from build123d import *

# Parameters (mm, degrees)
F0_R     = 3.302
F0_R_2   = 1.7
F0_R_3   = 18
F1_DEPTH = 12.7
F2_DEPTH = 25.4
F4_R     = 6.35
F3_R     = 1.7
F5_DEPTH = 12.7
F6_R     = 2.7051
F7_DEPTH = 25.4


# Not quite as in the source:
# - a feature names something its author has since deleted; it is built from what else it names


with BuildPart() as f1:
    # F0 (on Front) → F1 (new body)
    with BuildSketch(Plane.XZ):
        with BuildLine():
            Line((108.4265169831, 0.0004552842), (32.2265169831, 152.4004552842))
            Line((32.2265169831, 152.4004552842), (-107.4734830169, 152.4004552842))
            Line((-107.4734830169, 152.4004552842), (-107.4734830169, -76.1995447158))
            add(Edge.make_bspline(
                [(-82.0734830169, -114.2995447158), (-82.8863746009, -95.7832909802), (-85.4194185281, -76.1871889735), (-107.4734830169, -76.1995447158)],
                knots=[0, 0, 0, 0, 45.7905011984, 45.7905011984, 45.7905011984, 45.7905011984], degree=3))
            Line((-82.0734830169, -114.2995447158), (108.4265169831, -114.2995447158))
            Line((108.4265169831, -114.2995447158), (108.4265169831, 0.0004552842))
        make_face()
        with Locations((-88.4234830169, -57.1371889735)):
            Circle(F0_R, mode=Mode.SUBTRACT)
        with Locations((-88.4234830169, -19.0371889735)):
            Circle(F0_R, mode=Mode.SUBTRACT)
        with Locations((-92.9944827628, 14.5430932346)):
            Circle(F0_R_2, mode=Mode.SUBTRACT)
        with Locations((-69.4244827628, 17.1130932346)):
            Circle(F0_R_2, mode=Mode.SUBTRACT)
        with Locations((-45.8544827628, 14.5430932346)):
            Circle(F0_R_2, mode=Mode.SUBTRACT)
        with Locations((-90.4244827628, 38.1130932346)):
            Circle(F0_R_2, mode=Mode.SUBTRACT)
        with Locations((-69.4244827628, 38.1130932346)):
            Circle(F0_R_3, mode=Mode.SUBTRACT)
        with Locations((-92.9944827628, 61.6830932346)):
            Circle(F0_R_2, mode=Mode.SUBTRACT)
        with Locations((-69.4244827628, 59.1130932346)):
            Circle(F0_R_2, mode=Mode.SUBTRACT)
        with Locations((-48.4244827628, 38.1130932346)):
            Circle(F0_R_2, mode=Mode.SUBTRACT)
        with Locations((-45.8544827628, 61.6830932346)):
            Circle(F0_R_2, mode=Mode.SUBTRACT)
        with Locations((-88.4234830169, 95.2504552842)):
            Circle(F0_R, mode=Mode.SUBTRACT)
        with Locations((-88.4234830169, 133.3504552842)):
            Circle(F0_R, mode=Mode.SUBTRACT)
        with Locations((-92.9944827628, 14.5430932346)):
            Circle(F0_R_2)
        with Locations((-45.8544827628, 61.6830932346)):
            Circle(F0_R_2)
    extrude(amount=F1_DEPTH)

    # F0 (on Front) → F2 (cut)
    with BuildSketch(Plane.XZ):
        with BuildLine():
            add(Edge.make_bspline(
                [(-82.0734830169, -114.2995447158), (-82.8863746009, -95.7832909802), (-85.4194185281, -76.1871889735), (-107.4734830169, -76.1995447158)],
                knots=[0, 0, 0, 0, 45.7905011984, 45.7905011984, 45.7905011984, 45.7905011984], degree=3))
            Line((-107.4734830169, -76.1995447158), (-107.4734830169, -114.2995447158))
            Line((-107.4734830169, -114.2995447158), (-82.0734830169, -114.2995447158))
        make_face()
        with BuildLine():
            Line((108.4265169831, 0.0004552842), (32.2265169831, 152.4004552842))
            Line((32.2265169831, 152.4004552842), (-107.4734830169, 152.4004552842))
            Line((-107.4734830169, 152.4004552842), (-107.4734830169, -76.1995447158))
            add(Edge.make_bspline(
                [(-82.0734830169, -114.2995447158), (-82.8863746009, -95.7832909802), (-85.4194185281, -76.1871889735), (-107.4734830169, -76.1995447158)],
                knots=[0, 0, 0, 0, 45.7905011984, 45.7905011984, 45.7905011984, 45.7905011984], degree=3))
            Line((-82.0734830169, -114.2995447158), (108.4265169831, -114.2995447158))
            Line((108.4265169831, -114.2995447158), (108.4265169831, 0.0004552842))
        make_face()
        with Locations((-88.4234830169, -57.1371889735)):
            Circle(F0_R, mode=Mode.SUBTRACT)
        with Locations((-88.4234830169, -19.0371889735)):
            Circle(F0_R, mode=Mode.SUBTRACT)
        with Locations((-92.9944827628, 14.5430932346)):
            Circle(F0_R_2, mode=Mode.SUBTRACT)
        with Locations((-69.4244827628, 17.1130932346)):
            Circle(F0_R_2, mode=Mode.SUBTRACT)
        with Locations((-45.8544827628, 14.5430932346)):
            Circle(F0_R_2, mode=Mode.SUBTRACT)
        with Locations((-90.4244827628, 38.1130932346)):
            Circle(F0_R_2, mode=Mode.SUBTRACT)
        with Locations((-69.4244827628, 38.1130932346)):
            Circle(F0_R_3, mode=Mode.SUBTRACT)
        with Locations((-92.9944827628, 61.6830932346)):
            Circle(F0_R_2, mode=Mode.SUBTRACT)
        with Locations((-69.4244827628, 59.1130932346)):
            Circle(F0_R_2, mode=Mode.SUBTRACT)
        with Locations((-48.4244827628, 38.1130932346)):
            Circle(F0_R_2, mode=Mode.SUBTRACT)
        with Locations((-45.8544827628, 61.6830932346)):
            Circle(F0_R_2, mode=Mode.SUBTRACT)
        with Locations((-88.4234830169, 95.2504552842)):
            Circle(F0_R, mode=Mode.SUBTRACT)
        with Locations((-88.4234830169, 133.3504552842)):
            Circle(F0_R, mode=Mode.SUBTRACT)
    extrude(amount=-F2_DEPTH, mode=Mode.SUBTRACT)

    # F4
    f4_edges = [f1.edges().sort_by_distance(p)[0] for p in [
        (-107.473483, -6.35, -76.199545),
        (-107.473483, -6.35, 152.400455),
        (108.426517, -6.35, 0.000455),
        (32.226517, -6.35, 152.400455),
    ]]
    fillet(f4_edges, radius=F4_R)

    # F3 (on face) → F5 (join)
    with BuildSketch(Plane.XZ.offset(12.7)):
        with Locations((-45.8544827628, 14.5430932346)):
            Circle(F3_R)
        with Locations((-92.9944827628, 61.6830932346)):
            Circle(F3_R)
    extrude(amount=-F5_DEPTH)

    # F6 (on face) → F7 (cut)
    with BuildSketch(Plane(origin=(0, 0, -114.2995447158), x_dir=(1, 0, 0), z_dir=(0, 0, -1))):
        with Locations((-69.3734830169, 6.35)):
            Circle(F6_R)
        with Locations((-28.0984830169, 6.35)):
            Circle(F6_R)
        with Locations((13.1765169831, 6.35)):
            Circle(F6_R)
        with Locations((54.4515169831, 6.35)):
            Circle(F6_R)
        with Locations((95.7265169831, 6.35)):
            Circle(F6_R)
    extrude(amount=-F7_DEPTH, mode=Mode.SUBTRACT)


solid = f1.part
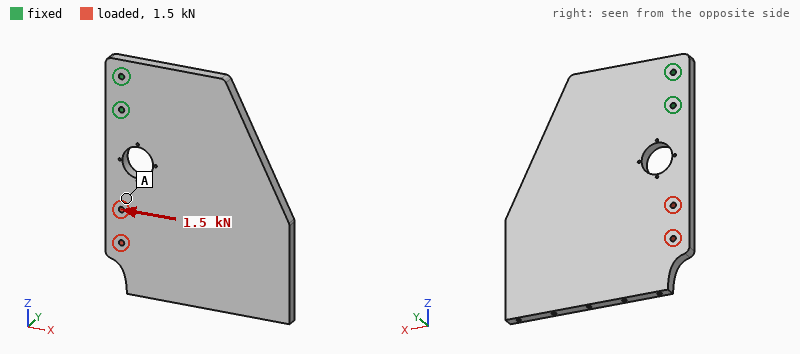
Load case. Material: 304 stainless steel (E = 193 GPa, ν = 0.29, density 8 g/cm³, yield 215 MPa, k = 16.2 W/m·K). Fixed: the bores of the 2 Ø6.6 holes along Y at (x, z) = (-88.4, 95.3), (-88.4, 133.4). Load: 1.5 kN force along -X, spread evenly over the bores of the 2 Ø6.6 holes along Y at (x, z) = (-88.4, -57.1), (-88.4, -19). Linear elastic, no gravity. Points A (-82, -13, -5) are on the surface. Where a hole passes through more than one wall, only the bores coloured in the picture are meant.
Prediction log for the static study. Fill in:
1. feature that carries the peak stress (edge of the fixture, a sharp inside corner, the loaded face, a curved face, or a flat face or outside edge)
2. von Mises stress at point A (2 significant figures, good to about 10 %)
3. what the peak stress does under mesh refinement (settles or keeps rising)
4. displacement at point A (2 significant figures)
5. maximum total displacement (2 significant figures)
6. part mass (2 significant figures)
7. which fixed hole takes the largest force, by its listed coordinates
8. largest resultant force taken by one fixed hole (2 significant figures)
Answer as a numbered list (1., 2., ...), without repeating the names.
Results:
1. edge of the fixture
2. 2.4 MPa
3. keeps rising
4. 18 µm
5. 45 µm
6. 5.0 kg
7. (-88.4, 95.3)
8. 6.2 kN
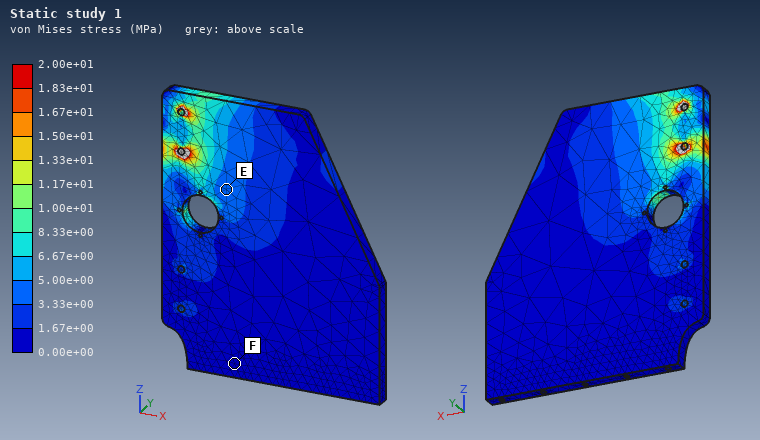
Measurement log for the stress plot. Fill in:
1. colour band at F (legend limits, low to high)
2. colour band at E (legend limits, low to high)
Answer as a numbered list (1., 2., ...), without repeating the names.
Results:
1. 0.00e+00 to 1.67e+00 MPa
2. 3.33e+00 to 5.00e+00 MPa
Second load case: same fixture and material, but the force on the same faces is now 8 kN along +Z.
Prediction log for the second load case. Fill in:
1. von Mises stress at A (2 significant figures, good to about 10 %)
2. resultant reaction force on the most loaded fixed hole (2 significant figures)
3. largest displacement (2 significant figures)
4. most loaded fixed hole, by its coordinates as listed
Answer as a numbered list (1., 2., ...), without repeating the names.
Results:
1. 10 MPa
2. 6.0 kN
3. 17 µm
4. (-88.4, 95.3)
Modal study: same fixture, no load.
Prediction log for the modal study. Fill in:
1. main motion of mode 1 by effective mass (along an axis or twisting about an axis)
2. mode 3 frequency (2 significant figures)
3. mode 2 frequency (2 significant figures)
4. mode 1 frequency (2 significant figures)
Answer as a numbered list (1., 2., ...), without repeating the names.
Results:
1. along Y
2. 550 Hz
3. 300 Hz
4. 120 Hz
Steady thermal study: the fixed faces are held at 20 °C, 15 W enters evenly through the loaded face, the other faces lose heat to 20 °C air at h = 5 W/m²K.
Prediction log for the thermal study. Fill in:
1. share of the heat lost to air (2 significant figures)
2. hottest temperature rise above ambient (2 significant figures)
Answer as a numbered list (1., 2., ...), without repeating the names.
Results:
1. 74 %
2. 62 K
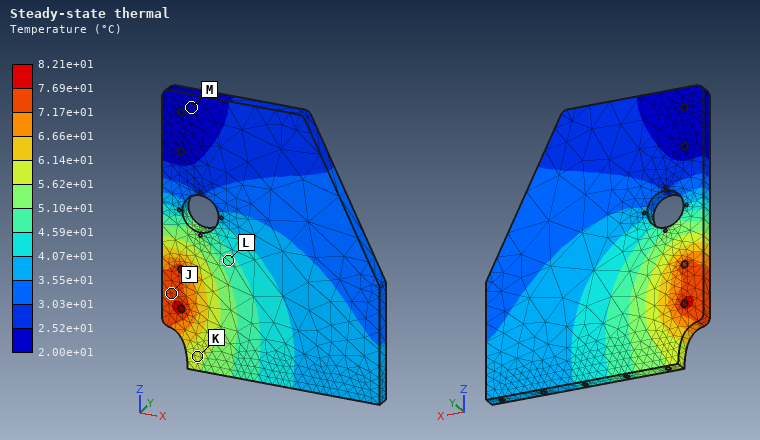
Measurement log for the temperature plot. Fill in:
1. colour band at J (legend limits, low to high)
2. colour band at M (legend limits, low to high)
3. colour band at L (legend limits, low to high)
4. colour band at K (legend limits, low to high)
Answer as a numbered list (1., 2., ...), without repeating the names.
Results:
1. 7.17e+01 to 7.69e+01 °C
2. 2.00e+01 to 2.52e+01 °C
3. 4.59e+01 to 5.10e+01 °C
4. 5.62e+01 to 6.14e+01 °C
